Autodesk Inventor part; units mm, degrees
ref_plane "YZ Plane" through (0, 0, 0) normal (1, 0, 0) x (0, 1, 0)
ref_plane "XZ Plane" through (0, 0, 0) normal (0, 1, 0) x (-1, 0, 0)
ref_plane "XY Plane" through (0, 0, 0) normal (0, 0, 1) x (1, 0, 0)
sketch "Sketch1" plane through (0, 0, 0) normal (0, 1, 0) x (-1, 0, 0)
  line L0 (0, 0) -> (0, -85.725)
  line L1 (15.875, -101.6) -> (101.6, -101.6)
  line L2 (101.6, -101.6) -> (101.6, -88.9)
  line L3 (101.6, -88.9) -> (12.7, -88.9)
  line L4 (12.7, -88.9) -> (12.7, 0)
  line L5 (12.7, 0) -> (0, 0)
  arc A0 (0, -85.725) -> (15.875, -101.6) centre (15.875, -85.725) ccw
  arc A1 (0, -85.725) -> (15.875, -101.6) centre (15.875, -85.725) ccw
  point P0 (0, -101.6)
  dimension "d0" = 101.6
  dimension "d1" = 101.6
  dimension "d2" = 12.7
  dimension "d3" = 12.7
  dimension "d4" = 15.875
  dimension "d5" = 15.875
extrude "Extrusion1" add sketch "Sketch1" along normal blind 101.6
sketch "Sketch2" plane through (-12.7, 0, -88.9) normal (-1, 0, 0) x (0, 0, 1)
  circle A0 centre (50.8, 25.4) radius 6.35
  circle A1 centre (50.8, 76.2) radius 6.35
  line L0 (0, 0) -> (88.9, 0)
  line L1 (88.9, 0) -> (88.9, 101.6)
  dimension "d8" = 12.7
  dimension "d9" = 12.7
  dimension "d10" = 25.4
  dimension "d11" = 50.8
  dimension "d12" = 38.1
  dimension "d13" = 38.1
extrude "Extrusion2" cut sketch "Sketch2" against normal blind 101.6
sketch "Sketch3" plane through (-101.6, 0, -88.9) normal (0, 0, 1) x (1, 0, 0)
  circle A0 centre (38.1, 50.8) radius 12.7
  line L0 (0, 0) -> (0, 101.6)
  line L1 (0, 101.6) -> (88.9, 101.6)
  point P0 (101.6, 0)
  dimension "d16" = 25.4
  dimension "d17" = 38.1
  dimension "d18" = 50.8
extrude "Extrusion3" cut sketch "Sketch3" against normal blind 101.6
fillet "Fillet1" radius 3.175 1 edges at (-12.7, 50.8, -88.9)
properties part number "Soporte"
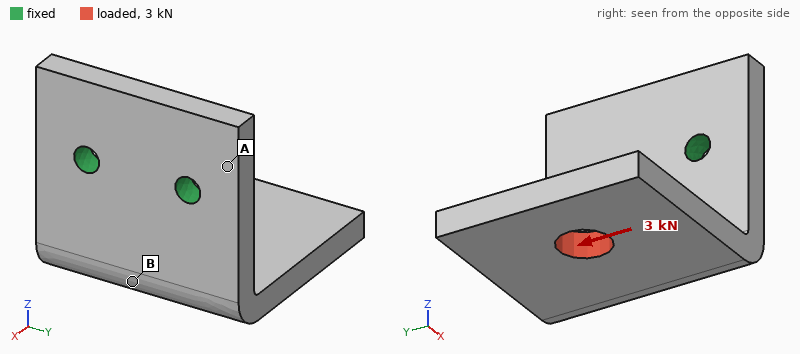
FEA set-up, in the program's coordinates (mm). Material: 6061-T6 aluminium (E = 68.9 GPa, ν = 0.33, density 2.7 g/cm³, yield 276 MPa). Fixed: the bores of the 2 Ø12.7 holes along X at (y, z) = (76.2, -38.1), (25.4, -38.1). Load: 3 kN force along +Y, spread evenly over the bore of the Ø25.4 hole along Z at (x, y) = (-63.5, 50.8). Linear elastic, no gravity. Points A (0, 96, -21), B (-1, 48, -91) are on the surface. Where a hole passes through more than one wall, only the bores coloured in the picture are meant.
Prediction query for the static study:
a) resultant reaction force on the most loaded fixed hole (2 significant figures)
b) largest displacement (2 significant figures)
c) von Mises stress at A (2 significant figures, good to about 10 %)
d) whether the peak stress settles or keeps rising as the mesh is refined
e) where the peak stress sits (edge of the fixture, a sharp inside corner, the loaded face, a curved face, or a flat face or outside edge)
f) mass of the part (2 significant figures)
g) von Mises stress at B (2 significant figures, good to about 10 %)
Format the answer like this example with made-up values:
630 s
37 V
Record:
4.1 kN
0.32 mm
8.1 MPa
keeps rising
edge of the fixture
620 g
21 MPa
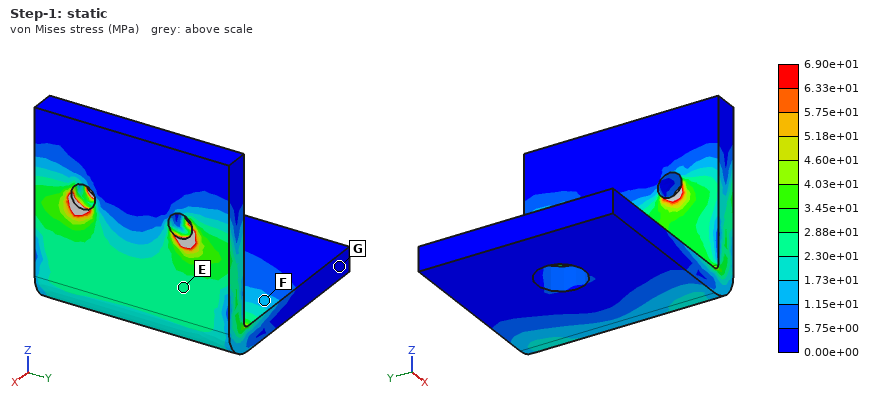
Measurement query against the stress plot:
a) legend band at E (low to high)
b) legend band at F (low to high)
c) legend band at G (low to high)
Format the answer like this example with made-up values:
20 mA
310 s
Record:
2.30e+01 to 2.88e+01 MPa
1.15e+01 to 1.73e+01 MPa
0.00e+00 to 5.75e+00 MPa
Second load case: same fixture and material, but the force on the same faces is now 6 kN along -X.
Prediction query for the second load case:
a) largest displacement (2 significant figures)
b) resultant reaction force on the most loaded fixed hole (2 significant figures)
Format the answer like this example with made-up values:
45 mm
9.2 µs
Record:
0.80 mm
3.0 kN
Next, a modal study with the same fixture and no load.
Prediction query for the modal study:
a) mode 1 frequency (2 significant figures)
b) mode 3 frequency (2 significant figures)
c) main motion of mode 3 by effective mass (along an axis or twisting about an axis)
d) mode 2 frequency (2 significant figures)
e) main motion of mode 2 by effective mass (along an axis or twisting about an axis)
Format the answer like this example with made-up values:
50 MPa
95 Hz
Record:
620 Hz
1900 Hz
along X
1100 Hz
along Y
